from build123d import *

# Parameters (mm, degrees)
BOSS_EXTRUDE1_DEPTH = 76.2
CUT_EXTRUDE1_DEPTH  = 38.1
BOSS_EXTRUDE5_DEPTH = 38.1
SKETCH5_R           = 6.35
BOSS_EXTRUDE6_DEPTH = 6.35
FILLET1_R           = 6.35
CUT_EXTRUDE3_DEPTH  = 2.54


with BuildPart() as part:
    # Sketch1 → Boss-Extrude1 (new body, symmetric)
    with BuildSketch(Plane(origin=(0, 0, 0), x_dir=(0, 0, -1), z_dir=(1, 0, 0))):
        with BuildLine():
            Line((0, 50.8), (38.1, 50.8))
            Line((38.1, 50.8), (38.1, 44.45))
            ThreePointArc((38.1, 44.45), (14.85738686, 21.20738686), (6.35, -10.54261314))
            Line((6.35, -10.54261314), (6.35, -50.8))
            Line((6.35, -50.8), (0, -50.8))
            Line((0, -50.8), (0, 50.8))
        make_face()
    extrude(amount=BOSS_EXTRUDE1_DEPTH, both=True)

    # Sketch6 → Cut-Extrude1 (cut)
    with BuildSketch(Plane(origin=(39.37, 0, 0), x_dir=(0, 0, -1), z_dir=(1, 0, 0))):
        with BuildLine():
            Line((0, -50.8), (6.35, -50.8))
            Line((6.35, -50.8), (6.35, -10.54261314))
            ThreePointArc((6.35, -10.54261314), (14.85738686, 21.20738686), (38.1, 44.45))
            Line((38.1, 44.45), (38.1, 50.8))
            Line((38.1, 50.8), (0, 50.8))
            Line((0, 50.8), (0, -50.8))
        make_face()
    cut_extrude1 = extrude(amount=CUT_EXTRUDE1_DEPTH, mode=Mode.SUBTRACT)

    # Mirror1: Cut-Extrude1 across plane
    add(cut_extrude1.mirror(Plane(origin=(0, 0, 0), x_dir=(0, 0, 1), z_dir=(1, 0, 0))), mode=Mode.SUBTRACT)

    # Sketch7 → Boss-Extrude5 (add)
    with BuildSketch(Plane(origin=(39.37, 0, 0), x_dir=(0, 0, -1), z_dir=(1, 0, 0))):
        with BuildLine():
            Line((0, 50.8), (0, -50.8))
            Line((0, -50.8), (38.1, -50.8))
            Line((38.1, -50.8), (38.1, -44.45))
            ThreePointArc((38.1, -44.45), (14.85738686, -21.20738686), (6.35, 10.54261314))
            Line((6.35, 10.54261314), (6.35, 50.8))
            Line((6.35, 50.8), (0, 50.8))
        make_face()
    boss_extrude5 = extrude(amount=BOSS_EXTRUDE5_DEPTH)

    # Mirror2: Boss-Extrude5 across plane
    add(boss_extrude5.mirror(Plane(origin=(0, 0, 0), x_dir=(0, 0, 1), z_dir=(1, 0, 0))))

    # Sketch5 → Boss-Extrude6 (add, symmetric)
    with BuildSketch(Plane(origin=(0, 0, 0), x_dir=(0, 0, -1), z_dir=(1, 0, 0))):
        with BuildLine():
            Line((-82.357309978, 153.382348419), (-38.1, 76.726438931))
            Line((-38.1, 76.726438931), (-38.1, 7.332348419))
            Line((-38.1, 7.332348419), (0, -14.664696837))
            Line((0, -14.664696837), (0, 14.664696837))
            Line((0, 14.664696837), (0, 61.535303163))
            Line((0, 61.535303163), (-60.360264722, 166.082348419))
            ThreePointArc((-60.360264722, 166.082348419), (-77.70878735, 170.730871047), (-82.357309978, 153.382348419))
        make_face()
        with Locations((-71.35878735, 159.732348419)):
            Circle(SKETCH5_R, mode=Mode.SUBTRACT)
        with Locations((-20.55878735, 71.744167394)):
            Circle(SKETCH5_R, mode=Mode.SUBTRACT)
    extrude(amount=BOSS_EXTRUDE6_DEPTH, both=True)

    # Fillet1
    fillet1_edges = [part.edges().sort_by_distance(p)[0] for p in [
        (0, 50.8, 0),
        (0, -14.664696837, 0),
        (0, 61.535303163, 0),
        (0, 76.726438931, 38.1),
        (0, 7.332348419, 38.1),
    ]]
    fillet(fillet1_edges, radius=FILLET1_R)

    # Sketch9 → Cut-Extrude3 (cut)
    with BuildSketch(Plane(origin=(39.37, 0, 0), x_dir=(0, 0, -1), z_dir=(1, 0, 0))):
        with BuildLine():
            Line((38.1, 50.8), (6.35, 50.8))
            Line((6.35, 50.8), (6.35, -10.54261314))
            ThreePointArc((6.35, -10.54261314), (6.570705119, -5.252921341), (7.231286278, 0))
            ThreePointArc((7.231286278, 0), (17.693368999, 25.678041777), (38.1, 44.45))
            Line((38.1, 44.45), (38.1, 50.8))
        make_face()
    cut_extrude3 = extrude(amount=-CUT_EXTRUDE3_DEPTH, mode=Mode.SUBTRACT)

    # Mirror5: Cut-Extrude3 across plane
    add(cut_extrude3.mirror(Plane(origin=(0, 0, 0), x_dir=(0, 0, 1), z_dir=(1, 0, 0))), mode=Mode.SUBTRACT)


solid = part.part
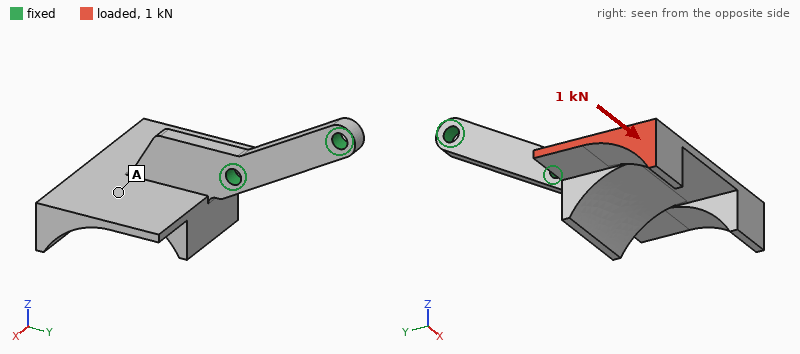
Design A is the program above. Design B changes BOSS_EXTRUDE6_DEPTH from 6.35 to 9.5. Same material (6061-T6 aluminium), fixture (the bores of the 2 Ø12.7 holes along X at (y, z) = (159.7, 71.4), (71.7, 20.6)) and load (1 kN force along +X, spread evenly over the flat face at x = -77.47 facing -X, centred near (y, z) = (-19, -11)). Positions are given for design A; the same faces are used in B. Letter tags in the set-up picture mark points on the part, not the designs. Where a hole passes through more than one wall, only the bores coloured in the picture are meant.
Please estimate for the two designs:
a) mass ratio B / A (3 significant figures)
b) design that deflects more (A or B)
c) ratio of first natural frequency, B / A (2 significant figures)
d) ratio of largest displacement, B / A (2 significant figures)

1.12
A
1.7
0.38
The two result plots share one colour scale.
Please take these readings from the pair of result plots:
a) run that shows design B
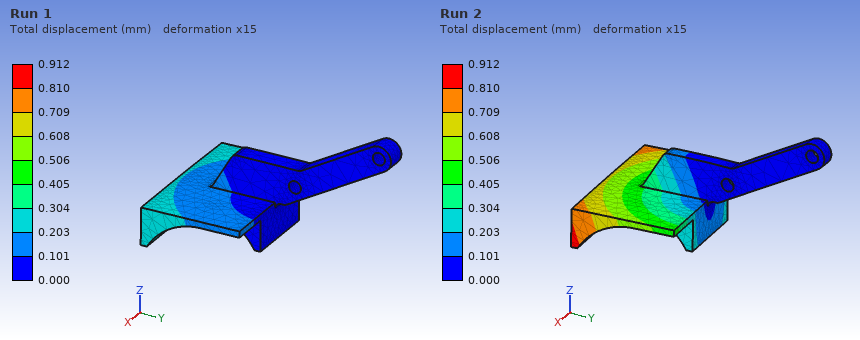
Run 1
